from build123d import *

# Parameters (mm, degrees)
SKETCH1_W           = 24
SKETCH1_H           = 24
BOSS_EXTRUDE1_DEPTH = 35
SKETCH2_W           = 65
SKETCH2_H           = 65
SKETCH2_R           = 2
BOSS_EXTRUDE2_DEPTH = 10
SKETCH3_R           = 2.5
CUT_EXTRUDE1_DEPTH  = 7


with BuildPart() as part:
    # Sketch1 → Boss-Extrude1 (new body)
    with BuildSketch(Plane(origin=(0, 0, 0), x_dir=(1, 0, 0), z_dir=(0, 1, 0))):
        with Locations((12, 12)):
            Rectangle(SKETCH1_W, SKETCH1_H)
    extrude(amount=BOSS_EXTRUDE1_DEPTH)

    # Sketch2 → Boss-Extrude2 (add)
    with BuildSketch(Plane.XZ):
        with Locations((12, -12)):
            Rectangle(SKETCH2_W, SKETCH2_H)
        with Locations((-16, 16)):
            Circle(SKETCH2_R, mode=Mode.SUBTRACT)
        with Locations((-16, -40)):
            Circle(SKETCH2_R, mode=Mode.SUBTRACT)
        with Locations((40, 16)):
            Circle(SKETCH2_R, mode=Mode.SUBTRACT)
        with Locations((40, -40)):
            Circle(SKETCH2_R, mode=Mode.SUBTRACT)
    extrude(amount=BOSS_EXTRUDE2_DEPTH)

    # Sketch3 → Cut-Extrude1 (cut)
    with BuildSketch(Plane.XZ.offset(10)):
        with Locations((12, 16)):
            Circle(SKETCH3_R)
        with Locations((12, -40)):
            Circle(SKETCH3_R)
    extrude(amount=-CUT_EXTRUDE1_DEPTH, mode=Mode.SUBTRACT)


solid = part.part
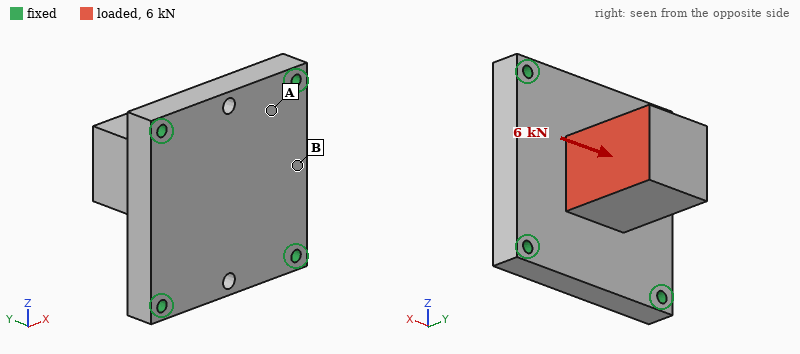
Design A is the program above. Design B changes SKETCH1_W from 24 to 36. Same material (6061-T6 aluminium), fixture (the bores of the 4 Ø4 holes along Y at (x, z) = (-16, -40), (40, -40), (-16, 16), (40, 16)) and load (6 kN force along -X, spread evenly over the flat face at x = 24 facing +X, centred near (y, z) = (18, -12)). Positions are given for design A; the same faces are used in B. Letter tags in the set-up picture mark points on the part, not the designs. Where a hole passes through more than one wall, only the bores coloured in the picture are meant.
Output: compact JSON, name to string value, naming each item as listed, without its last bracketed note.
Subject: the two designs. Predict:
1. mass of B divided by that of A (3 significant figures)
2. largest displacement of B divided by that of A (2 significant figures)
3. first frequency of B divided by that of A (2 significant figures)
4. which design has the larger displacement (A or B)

{"mass of B divided by that of A": "1.16", "largest displacement of B divided by that of A": "0.62", "first frequency of B divided by that of A": "0.96", "which design has the larger displacement": "A"}
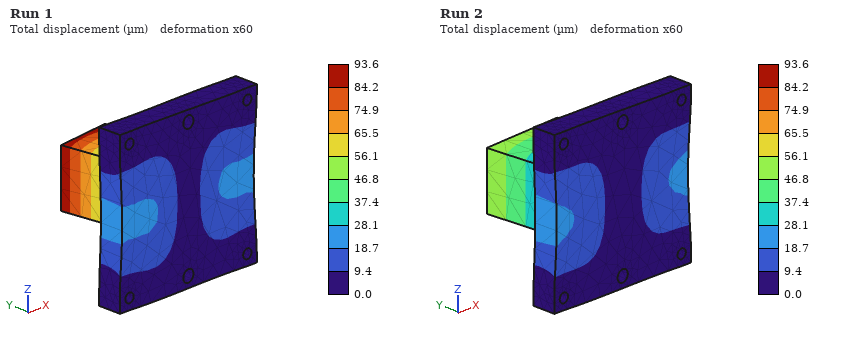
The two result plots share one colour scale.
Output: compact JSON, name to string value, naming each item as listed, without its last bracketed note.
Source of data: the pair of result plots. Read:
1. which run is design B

{"which run is design B": "Run 2"}
